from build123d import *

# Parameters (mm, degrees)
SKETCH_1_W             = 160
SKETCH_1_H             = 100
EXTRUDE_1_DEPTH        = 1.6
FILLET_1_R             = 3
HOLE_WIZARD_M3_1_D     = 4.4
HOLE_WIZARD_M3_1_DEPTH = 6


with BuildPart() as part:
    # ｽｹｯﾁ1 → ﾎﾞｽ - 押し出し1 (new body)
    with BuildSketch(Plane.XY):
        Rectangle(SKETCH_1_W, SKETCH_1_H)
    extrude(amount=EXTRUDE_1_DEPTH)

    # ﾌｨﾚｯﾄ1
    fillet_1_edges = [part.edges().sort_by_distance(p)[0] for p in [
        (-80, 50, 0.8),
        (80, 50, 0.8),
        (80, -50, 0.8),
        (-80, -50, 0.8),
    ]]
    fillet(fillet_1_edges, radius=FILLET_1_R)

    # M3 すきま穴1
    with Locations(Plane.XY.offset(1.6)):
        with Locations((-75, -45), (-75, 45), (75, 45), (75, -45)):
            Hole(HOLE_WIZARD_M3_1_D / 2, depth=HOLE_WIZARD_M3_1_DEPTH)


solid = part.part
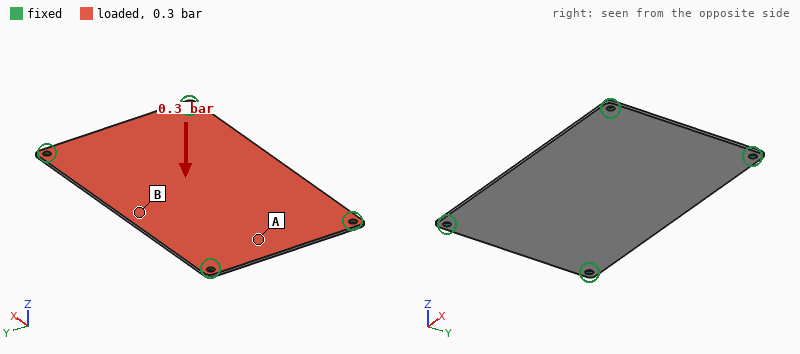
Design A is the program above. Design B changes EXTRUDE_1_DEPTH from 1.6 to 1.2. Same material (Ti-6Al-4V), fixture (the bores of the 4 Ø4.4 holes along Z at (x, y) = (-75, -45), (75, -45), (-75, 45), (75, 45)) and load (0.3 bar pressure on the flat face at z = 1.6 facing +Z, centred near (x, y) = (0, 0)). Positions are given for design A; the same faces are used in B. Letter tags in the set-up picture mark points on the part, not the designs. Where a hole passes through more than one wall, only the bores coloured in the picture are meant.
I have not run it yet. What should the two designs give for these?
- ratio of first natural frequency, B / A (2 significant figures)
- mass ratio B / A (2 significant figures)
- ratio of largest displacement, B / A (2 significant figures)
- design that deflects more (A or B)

0.75
0.75
2.3
B
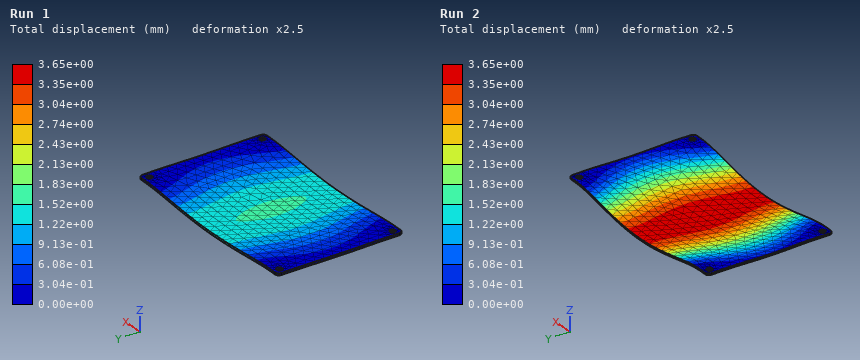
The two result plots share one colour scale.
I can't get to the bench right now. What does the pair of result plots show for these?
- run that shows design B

Run 2
